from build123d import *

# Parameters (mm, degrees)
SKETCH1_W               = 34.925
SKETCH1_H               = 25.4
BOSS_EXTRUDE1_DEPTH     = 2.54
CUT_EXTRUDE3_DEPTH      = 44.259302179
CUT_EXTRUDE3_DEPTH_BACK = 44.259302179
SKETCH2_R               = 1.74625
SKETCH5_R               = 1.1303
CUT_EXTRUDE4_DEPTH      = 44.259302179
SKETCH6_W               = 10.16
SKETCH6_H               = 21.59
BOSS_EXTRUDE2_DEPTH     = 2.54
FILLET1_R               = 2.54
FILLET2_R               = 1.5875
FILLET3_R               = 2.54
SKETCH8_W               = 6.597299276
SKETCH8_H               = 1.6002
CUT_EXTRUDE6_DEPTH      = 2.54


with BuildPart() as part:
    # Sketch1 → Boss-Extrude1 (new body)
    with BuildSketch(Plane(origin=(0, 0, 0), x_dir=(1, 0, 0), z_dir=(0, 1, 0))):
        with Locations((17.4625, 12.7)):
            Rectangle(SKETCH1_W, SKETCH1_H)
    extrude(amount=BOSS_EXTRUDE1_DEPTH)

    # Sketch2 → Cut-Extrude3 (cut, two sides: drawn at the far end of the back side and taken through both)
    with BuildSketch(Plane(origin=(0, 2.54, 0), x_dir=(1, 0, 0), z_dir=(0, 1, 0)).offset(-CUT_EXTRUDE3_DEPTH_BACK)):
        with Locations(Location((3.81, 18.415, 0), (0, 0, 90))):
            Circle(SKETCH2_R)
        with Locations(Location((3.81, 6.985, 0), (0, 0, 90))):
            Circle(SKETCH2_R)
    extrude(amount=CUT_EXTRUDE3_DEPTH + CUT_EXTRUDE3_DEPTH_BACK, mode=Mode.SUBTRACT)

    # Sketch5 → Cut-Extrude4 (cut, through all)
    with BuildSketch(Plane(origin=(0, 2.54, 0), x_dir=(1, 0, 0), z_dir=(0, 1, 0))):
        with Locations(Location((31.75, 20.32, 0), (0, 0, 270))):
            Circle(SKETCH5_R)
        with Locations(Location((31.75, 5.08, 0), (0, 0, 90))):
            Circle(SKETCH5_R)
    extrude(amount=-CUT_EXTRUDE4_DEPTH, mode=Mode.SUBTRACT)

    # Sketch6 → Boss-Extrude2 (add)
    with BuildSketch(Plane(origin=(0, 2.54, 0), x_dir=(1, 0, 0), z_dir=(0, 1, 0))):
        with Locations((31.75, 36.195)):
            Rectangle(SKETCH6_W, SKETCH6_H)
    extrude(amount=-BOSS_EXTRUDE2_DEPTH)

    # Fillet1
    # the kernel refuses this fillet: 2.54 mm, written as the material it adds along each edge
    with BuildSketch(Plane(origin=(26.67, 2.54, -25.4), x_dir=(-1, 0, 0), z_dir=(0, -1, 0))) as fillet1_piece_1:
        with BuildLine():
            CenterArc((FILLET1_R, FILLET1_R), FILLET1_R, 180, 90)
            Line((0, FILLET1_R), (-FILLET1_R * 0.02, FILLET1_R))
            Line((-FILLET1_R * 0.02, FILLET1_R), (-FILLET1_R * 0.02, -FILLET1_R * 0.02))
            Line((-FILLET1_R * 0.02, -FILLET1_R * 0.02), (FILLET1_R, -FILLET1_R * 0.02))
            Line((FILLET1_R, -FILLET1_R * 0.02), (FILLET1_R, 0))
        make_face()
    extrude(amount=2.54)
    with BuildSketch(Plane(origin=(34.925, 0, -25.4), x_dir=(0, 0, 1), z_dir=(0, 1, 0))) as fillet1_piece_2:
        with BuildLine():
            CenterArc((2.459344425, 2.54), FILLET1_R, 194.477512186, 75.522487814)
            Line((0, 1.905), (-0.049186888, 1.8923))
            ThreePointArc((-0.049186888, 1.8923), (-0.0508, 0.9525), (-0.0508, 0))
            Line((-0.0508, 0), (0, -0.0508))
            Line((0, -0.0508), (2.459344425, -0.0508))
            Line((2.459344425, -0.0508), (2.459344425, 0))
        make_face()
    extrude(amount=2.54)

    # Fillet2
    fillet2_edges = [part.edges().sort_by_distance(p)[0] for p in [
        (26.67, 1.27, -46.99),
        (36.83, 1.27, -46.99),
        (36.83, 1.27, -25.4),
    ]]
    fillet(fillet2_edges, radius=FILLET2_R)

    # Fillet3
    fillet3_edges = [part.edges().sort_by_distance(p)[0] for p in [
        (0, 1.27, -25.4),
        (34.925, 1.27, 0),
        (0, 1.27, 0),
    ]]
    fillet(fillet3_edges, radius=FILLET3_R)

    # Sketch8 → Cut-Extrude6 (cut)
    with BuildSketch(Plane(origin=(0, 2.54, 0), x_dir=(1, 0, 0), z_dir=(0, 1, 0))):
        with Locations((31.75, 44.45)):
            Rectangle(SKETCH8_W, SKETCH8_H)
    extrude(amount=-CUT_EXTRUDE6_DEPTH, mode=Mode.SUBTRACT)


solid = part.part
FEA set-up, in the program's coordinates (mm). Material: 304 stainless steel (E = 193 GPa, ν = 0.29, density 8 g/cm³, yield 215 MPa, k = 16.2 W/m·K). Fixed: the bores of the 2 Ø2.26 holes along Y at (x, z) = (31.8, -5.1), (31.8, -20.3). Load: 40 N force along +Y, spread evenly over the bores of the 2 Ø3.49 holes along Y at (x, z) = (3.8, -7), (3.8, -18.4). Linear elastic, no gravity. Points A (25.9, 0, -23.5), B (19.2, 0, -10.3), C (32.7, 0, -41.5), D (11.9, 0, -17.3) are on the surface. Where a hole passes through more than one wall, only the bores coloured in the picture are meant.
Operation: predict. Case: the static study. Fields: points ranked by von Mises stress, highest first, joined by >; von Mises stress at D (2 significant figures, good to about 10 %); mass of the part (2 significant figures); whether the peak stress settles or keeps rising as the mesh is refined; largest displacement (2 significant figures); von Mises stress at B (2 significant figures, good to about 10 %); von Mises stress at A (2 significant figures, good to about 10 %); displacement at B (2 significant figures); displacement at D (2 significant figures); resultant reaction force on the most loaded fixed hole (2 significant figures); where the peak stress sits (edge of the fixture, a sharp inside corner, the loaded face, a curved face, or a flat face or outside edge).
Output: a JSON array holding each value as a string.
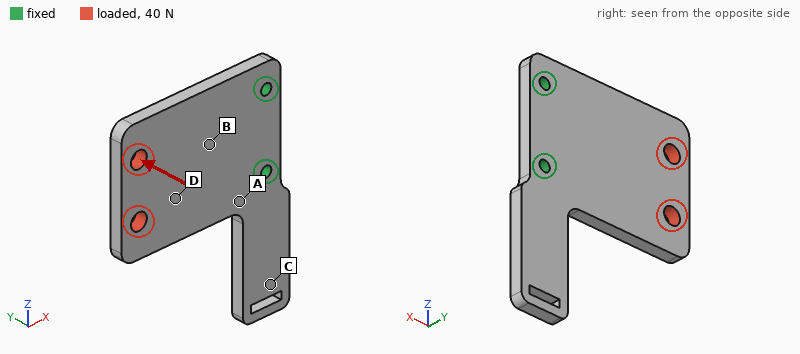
["A > B > D > C", "13 MPa", "22 g", "keeps rising", "54 µm", "21 MPa", "33 MPa", "13 µm", "26 µm", "20 N", "edge of the fixture"]
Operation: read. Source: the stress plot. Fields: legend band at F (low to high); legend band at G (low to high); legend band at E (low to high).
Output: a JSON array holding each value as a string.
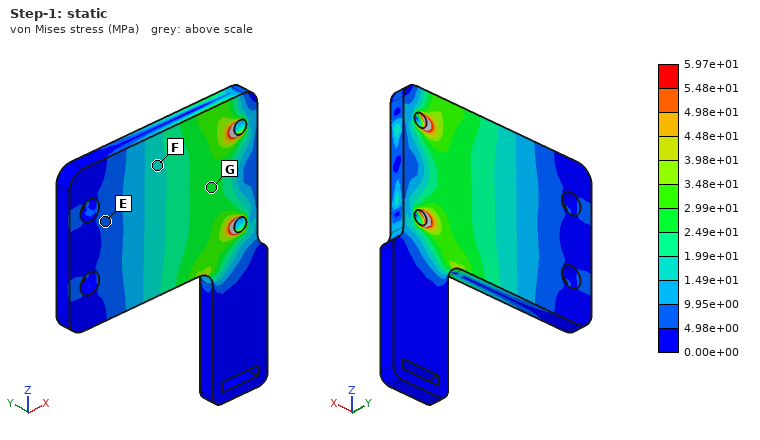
["1.49e+01 to 1.99e+01 MPa", "2.49e+01 to 2.99e+01 MPa", "4.98e+00 to 9.95e+00 MPa"]
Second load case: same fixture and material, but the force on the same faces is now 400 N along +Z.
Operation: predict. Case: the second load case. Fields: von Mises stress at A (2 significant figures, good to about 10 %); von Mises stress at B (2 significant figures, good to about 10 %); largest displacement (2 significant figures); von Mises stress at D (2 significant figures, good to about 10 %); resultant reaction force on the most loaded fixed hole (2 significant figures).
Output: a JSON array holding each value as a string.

["23 MPa", "17 MPa", "11 µm", "15 MPa", "700 N"]
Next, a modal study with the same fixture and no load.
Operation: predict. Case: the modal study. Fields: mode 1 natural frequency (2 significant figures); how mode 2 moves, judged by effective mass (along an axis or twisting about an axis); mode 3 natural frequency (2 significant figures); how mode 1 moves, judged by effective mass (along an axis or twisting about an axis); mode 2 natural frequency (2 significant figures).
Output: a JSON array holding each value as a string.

["2000 Hz", "along Y", "5800 Hz", "along Y", "3100 Hz"]
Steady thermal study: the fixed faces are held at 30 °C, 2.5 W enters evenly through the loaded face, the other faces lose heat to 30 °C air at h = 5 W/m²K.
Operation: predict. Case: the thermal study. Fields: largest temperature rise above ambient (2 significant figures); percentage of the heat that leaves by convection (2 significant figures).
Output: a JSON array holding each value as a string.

["69 K", "14 %"]
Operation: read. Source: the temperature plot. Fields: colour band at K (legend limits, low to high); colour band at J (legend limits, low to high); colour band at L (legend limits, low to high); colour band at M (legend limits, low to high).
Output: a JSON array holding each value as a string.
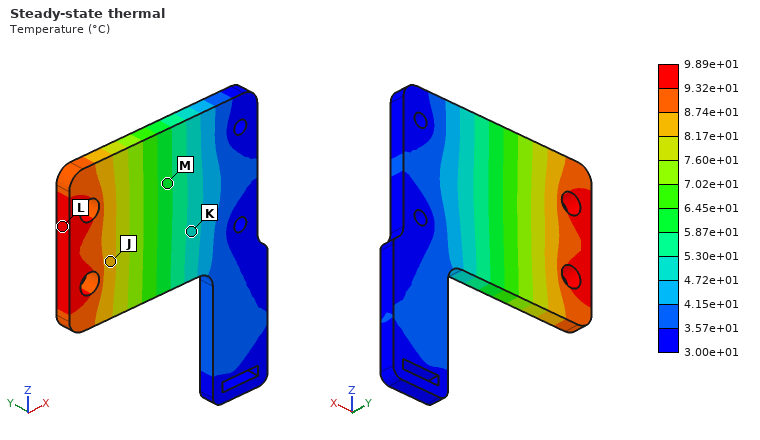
["4.72e+01 to 5.30e+01 °C", "8.17e+01 to 8.74e+01 °C", "9.32e+01 to 9.89e+01 °C", "5.87e+01 to 6.45e+01 °C"]
